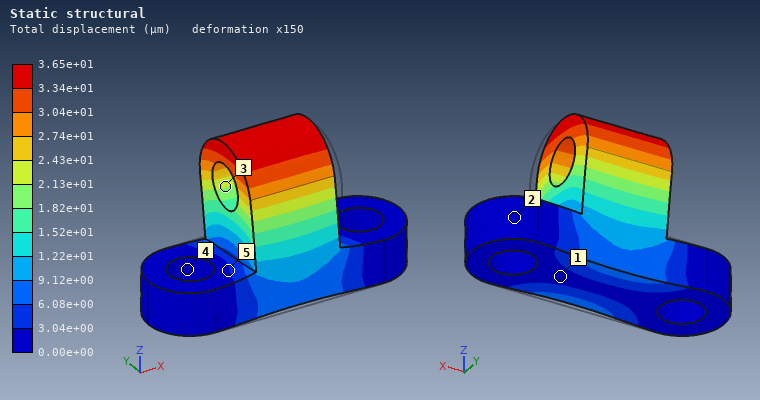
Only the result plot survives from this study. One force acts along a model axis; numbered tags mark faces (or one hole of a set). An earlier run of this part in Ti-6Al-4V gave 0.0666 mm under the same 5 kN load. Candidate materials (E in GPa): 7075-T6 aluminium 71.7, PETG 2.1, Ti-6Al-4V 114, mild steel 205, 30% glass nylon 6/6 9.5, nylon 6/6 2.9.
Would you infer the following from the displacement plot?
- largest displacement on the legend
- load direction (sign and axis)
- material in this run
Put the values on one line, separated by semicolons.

3.65e+01 µm; +Y; mild steel
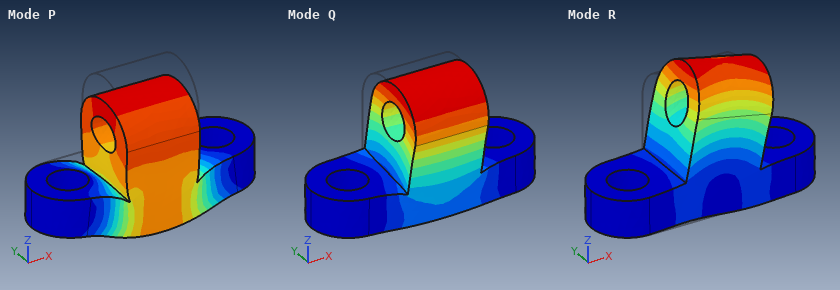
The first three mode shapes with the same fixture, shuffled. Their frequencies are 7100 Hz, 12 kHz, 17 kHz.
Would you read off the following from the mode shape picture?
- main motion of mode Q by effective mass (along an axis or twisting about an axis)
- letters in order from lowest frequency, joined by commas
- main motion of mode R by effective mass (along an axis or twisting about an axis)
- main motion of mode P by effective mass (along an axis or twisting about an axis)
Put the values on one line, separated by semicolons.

along Y; Q, R, P; along X; along Z
